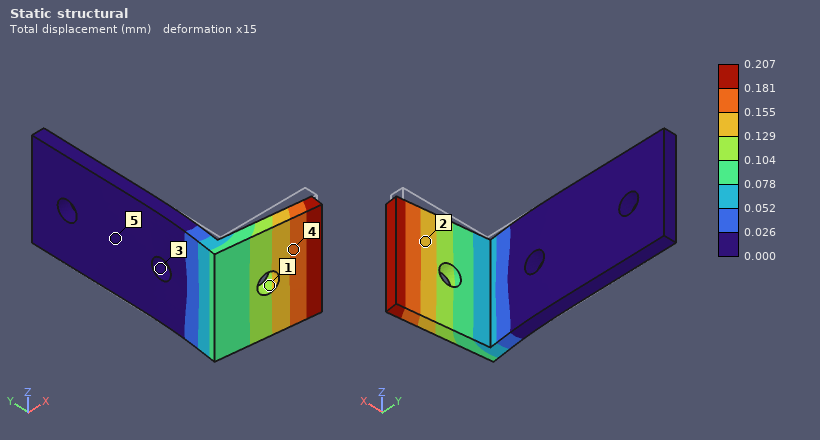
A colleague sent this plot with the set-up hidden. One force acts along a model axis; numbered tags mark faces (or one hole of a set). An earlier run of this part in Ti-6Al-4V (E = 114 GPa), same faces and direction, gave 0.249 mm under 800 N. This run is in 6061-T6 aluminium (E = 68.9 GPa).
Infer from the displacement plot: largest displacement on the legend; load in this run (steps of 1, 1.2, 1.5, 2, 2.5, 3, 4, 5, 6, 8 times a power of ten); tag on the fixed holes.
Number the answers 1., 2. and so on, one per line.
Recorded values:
1. 0.207 mm
2. 400 N
3. 3
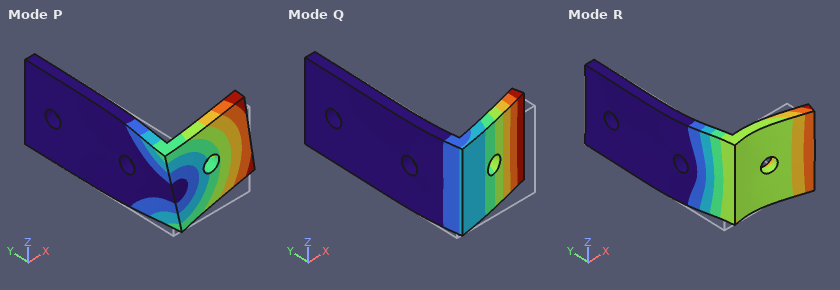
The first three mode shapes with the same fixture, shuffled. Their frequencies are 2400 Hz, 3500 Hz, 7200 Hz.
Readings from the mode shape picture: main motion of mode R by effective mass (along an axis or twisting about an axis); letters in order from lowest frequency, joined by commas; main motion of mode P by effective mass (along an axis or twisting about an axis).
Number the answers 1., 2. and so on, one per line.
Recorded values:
1. along X
2. Q, P, R
3. along Z
